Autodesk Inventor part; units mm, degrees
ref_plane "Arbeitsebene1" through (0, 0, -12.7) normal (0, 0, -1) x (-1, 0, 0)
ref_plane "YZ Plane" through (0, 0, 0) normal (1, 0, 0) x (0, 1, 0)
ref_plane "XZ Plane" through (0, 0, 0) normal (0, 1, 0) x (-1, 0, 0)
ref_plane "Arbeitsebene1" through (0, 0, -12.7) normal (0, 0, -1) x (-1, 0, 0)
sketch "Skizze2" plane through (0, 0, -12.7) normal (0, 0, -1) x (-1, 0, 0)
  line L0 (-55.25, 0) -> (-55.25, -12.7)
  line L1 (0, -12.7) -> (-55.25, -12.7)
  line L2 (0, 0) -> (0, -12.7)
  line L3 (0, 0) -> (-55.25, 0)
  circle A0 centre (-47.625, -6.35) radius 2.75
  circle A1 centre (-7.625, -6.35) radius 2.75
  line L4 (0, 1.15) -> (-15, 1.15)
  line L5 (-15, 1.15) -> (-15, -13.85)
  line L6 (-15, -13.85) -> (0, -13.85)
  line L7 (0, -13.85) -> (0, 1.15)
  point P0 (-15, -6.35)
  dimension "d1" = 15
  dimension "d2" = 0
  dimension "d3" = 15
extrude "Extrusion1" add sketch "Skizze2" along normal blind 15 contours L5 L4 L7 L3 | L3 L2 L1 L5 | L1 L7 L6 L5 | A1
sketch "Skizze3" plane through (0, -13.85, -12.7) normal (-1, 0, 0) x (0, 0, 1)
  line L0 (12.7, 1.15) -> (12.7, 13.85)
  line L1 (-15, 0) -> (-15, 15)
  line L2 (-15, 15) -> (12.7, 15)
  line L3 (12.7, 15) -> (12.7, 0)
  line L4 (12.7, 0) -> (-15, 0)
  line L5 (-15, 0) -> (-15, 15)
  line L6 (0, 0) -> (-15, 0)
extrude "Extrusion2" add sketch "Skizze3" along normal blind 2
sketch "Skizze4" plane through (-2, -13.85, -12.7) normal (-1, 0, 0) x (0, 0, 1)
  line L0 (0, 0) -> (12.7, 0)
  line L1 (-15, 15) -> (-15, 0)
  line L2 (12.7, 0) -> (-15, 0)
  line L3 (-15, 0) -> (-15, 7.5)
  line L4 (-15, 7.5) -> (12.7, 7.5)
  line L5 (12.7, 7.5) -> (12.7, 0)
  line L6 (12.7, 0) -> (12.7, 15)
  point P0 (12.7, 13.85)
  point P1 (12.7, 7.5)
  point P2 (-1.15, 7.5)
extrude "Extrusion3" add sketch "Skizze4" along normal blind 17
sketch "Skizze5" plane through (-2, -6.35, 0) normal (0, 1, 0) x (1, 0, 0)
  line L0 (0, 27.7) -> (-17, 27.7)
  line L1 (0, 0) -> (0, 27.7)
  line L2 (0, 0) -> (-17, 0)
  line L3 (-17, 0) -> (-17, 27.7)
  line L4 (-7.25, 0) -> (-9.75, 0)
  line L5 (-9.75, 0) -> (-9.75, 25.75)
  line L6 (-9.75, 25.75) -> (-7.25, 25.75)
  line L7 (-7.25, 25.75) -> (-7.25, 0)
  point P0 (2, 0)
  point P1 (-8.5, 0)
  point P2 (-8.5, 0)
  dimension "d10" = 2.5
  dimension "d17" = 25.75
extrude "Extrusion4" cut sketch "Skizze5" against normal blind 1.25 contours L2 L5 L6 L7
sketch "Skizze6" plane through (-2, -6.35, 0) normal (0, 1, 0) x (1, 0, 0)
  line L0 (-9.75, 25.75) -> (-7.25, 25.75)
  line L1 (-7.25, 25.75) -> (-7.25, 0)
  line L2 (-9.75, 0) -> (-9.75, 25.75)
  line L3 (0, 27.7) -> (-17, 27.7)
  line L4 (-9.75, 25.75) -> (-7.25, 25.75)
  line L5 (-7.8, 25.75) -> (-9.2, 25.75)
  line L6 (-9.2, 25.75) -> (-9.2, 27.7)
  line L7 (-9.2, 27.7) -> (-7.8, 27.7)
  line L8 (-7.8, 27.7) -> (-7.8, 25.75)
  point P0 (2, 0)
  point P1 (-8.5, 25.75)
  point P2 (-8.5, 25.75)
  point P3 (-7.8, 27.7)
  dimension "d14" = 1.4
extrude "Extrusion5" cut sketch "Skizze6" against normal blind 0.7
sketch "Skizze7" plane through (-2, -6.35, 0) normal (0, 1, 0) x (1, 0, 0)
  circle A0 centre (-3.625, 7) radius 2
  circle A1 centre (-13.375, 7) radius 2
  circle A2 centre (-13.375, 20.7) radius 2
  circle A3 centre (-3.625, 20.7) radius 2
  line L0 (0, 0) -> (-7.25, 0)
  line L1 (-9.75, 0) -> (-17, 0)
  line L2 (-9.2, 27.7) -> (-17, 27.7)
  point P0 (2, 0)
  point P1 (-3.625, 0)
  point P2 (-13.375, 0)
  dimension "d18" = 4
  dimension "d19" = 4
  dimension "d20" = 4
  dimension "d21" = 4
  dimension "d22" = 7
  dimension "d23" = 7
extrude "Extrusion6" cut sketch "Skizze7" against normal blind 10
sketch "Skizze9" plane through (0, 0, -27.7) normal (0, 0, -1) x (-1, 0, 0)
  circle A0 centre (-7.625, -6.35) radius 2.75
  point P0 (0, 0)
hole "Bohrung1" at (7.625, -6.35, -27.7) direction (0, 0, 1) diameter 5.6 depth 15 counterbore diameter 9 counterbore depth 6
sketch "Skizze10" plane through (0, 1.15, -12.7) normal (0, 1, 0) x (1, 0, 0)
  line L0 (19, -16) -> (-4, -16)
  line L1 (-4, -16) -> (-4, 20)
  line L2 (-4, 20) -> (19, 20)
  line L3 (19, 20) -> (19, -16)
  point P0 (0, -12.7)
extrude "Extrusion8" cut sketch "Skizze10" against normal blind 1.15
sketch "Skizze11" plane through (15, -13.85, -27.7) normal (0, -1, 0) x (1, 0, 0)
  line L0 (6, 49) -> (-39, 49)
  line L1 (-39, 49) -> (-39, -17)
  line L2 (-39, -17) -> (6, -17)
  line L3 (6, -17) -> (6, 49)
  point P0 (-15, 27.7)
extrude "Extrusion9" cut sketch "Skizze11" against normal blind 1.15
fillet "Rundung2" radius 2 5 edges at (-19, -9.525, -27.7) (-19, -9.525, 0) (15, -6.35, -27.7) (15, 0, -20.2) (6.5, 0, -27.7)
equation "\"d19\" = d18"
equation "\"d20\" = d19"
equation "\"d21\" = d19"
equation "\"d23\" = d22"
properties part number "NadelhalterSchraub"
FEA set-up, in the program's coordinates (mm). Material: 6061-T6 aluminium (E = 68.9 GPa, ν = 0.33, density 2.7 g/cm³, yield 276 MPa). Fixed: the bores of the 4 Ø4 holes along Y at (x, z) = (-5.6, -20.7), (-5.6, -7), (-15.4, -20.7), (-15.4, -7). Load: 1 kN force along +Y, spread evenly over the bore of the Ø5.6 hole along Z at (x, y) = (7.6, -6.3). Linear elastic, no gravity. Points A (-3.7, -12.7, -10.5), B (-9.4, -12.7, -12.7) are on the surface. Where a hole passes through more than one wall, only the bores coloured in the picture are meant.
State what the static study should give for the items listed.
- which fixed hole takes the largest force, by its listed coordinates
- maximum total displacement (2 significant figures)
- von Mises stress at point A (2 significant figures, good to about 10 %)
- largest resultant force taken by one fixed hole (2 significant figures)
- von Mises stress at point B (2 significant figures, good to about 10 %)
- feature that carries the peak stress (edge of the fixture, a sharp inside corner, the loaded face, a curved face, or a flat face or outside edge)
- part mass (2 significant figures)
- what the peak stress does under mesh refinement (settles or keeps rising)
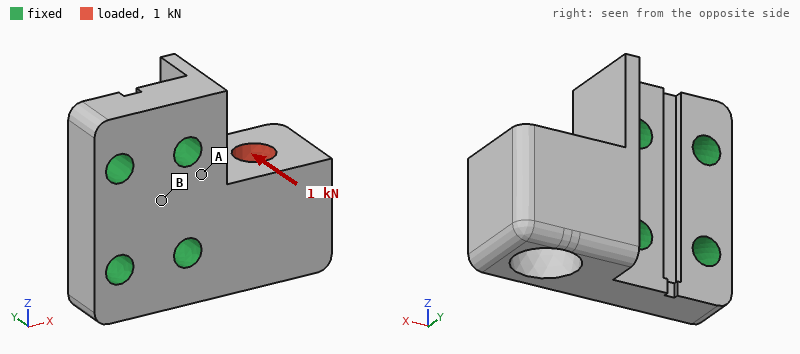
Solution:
(-5.6, -20.7)
58 µm
46 MPa
900 N
15 MPa
edge of the fixture
15 g
keeps rising
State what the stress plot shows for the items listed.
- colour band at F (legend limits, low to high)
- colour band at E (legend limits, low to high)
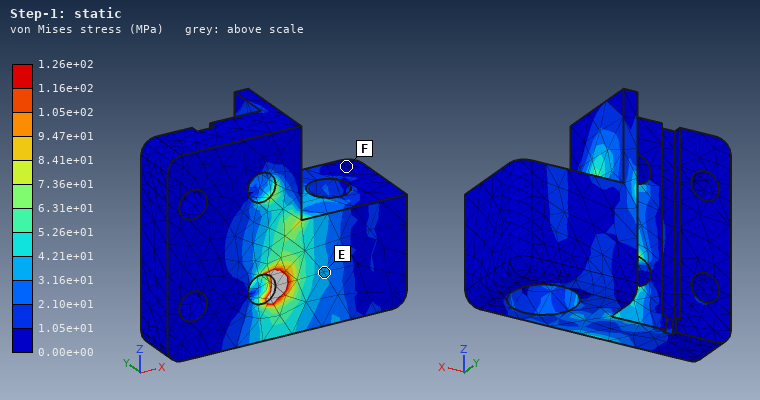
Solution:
0.00e+00 to 1.05e+01 MPa
3.16e+01 to 4.21e+01 MPa
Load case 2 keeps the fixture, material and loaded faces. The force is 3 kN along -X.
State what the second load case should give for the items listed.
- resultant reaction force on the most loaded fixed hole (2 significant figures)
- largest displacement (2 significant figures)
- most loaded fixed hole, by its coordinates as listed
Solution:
2.0 kN
50 µm
(-5.6, -20.7)
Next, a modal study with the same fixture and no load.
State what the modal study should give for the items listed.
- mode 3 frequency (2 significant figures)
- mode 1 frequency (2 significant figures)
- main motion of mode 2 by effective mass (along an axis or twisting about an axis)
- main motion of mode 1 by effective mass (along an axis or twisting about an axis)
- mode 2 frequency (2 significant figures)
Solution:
28 kHz
9800 Hz
along Z
along Y
18 kHz
